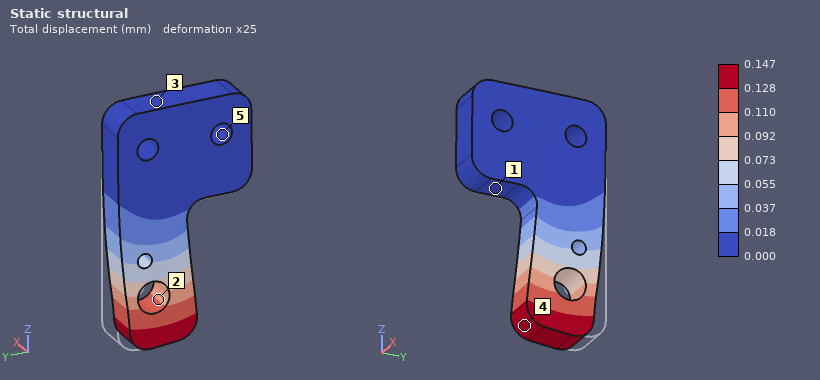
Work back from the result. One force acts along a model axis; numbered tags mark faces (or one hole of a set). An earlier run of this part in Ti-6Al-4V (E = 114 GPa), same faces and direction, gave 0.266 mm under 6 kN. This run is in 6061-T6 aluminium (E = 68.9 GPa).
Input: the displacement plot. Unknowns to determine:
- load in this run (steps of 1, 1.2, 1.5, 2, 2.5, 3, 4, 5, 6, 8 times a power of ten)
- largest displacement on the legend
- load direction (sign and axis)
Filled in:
2 kN
0.147 mm
-Y
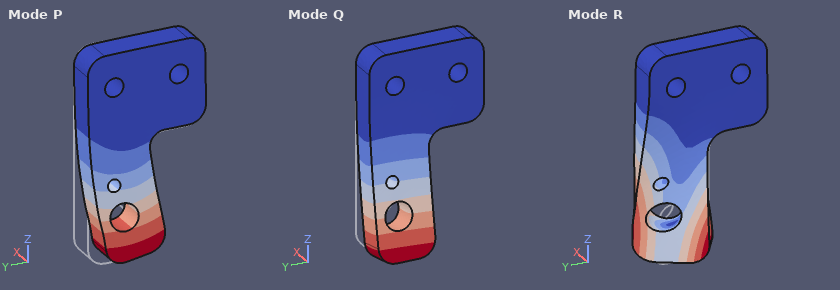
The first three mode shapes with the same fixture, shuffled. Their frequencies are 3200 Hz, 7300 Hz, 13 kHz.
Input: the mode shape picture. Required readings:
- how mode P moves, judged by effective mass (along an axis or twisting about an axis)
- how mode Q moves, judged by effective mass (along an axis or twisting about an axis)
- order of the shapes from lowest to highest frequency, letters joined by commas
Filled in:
along Y
along X
Q, P, R
